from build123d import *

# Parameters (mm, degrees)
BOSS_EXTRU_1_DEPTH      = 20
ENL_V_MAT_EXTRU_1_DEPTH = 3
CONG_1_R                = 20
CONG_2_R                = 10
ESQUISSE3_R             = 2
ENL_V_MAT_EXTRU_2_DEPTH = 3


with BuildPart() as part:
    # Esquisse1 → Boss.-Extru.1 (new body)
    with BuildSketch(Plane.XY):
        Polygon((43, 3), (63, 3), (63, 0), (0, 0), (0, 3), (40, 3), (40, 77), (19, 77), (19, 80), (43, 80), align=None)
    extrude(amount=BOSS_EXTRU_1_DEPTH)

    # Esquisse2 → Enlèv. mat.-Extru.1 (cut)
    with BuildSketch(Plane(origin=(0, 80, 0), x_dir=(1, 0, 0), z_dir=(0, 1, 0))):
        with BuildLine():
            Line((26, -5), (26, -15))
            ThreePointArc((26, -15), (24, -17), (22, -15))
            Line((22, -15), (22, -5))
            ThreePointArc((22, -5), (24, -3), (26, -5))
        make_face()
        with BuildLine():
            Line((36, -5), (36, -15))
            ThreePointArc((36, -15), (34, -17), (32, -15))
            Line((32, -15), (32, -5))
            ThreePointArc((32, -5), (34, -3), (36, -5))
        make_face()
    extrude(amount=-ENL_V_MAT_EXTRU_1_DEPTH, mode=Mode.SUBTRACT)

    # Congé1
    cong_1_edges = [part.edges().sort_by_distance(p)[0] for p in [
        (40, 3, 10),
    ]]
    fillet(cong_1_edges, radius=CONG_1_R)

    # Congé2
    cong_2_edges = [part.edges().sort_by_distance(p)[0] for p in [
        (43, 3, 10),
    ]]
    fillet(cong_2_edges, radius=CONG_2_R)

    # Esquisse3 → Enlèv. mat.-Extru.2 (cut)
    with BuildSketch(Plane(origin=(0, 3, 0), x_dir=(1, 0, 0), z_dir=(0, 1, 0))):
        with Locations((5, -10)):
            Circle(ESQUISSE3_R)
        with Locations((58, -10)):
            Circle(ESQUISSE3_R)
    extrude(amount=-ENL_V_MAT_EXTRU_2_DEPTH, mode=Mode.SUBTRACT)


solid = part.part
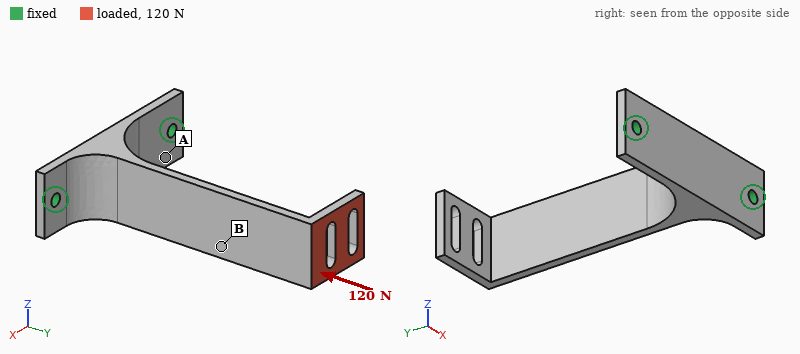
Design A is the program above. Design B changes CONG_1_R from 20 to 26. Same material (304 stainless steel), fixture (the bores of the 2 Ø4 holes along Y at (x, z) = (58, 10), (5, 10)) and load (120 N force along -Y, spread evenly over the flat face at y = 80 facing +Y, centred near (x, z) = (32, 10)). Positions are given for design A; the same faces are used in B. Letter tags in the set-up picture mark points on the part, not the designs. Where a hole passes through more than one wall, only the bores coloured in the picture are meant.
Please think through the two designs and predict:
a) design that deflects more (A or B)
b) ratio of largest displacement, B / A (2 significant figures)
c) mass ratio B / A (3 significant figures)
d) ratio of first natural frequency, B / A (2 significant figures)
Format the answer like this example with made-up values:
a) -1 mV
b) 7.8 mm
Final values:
a) A
b) 0.87
c) 1.10
d) 1.2
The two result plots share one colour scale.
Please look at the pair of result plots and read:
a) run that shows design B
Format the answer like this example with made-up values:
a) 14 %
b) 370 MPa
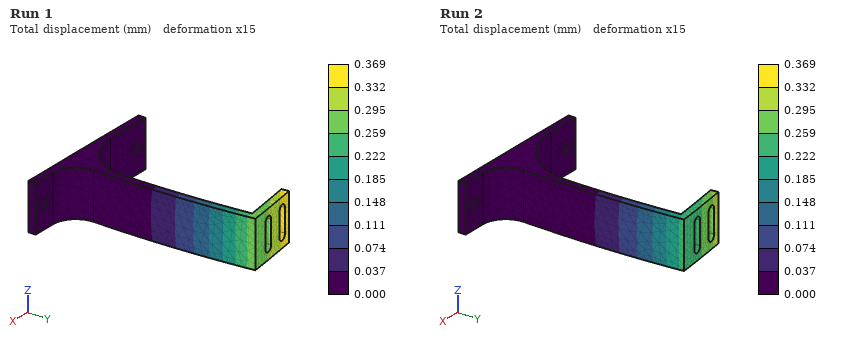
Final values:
a) Run 2
